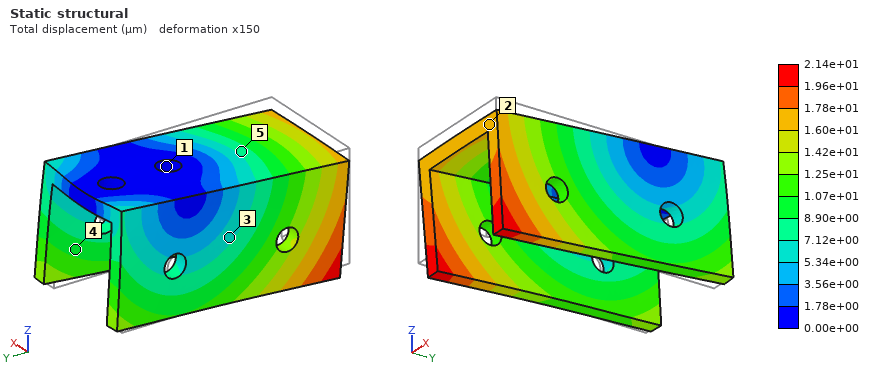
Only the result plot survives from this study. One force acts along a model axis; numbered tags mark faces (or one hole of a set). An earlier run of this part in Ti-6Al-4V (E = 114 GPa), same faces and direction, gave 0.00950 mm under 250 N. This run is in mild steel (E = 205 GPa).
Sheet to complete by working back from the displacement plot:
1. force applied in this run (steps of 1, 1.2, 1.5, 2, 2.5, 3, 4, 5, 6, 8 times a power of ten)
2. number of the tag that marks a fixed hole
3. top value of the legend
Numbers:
1 kN
1
2.14e+01 µm
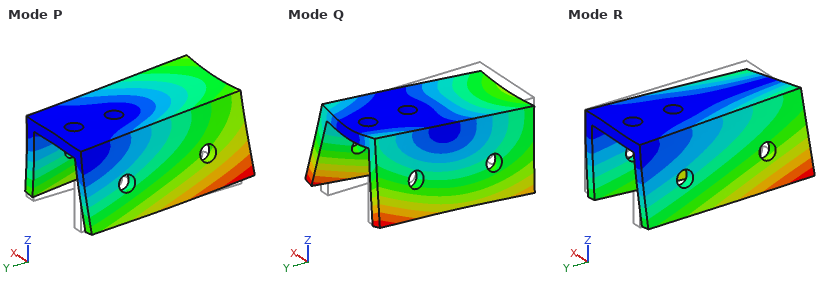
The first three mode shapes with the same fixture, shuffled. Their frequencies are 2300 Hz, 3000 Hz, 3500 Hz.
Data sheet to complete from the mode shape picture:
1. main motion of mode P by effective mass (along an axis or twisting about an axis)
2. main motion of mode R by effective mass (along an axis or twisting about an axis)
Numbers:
along Z
along X
